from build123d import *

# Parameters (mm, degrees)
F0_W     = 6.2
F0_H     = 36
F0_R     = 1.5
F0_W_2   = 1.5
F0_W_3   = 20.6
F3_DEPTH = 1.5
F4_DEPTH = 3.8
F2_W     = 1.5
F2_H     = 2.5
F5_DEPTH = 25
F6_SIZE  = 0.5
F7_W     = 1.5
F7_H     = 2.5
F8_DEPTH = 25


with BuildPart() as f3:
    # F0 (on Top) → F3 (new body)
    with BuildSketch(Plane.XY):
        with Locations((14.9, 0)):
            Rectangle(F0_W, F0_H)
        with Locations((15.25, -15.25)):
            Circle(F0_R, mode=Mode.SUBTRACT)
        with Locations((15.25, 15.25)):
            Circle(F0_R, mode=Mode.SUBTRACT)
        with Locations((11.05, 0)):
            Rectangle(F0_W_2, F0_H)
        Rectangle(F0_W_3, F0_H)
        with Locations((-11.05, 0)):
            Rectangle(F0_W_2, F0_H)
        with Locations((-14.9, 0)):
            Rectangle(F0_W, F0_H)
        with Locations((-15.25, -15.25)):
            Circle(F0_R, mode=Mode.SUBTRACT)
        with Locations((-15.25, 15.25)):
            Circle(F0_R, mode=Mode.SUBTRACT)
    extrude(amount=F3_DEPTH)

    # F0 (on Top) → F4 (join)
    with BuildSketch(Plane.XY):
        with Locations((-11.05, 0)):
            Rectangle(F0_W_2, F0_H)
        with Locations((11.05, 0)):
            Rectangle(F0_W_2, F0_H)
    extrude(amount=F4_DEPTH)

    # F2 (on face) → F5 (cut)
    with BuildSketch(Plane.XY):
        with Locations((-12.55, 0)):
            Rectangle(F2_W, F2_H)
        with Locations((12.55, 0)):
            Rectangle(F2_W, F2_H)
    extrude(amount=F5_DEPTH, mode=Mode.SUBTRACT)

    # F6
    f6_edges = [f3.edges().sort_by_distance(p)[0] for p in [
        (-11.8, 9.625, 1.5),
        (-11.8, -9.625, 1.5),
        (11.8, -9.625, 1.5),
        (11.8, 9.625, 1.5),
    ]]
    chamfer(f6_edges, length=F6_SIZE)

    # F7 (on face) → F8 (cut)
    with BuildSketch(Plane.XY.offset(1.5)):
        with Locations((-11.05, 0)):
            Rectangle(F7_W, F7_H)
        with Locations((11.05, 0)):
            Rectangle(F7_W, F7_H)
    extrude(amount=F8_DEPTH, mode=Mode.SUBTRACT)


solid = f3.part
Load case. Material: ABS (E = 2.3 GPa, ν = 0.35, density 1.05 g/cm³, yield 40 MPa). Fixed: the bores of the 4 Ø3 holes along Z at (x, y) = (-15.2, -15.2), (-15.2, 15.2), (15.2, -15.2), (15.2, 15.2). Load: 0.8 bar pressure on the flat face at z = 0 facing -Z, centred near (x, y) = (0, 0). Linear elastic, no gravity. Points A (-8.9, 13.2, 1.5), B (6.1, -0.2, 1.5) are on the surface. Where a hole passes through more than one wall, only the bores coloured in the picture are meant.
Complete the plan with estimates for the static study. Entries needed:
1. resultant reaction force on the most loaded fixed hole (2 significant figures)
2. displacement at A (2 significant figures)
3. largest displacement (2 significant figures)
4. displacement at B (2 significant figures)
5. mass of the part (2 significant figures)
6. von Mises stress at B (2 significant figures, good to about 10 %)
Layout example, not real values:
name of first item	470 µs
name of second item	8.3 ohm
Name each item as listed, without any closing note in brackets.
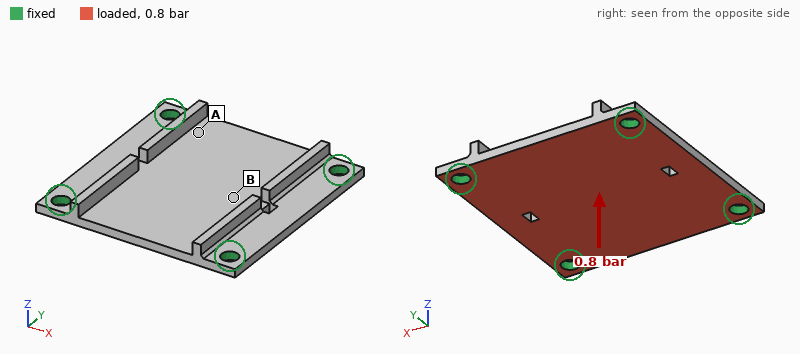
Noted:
resultant reaction force on the most loaded fixed hole	25 N
displacement at A	0.17 mm
largest displacement	0.53 mm
displacement at B	0.47 mm
mass of the part	2.2 g
von Mises stress at B	8.5 MPa
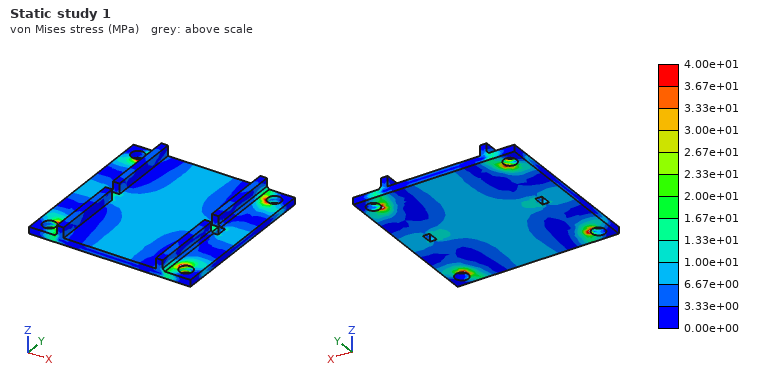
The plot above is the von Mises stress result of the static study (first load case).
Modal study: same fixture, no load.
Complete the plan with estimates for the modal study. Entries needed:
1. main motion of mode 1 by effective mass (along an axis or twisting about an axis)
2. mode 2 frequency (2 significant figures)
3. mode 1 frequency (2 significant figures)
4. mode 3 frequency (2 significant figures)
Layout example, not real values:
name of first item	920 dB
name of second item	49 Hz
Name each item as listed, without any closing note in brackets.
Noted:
main motion of mode 1 by effective mass	along Z
mode 2 frequency	3100 Hz
mode 1 frequency	1900 Hz
mode 3 frequency	3100 Hz
